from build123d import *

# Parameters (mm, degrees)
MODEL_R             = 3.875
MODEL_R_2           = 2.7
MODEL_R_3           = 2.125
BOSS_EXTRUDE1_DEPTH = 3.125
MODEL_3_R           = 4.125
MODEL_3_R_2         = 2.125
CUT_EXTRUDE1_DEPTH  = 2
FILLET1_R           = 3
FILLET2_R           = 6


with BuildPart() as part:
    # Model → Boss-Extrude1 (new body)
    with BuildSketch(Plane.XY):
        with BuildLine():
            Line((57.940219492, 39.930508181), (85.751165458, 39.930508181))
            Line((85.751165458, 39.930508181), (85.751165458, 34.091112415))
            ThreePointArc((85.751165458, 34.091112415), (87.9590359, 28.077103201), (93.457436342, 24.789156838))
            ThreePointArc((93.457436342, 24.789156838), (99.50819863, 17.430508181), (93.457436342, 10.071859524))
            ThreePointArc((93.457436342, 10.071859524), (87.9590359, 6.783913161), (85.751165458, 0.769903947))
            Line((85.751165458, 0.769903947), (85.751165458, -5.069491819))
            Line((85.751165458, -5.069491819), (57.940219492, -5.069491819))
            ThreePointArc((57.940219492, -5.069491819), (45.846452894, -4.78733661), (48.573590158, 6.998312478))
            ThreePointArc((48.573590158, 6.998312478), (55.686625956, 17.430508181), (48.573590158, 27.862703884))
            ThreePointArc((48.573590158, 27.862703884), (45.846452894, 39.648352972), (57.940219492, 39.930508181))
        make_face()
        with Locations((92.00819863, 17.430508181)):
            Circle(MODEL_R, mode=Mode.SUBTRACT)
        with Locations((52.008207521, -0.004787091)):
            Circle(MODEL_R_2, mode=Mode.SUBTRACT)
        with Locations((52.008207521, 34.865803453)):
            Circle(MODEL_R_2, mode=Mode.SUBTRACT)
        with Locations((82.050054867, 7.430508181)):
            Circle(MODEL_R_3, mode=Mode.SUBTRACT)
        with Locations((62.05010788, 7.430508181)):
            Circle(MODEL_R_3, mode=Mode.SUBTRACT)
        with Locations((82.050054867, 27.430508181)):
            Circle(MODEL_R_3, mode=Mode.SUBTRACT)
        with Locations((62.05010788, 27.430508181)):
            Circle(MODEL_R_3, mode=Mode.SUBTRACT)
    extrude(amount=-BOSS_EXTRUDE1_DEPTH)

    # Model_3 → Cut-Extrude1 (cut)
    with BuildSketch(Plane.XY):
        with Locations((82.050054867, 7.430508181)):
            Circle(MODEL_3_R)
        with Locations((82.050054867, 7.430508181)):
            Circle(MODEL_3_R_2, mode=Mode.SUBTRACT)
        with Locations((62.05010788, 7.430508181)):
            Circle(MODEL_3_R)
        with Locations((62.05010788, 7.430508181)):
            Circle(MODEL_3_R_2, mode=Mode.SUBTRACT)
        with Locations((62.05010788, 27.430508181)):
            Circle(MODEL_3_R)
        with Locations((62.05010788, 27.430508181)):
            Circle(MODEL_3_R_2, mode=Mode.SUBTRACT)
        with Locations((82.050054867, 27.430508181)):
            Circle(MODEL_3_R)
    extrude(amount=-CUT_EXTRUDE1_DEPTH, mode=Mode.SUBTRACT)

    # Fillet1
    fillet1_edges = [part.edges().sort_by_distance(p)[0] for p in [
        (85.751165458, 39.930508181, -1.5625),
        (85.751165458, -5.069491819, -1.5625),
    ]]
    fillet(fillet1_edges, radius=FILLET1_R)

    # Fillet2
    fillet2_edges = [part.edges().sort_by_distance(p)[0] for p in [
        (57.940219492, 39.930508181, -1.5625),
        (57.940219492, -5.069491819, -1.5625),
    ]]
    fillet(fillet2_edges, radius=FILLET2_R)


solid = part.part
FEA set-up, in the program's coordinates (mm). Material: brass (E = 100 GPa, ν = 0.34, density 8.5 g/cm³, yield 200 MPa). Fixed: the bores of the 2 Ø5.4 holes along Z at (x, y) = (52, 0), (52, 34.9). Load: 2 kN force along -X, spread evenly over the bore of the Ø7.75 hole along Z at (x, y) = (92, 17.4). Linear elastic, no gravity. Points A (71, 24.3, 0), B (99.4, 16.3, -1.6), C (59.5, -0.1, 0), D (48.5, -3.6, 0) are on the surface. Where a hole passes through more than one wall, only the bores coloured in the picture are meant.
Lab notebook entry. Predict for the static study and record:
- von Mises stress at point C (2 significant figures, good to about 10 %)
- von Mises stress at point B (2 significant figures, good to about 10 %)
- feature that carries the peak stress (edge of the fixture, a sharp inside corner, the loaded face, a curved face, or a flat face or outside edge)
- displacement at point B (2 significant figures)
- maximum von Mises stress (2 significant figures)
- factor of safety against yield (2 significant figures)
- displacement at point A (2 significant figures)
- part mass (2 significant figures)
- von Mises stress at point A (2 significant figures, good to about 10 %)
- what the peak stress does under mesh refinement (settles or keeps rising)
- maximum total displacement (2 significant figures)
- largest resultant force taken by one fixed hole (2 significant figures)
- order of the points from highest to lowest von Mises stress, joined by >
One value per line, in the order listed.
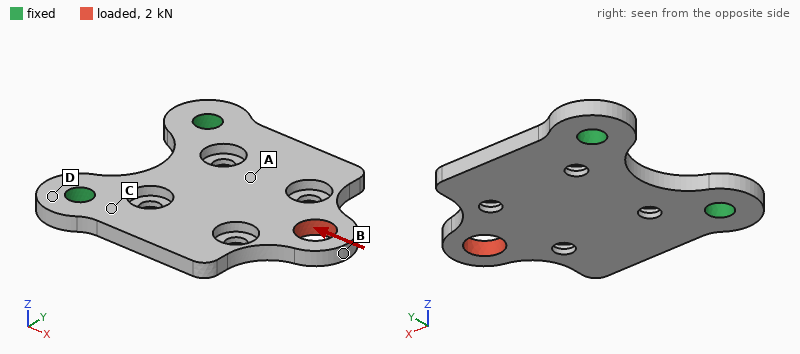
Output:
33 MPa
46 MPa
a curved face
35 µm
120 MPa
1.7
7.7 µm
44 g
19 MPa
settles
37 µm
1.1 kN
B > C > A > D
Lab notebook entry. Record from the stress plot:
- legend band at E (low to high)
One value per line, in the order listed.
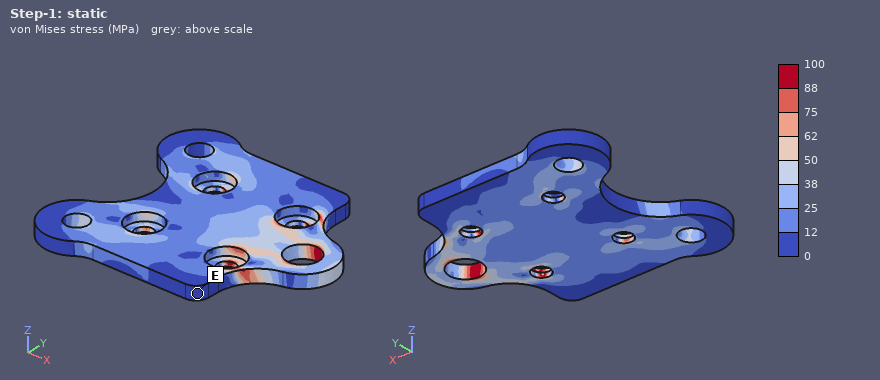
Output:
0 to 12 MPa
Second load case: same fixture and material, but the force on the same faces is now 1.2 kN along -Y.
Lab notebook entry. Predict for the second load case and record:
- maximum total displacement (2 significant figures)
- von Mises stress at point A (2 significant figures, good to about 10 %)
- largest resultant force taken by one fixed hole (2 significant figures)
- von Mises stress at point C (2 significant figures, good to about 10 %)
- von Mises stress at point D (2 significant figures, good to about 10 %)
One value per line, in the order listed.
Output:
43 µm
24 MPa
1.4 kN
38 MPa
13 MPa
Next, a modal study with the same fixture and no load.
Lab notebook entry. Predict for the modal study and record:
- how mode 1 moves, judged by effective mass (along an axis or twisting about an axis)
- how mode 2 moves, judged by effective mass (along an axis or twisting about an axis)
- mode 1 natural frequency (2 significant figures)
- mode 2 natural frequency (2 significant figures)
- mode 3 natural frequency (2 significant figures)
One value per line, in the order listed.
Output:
along Z
twisting about X
1100 Hz
3100 Hz
4800 Hz
